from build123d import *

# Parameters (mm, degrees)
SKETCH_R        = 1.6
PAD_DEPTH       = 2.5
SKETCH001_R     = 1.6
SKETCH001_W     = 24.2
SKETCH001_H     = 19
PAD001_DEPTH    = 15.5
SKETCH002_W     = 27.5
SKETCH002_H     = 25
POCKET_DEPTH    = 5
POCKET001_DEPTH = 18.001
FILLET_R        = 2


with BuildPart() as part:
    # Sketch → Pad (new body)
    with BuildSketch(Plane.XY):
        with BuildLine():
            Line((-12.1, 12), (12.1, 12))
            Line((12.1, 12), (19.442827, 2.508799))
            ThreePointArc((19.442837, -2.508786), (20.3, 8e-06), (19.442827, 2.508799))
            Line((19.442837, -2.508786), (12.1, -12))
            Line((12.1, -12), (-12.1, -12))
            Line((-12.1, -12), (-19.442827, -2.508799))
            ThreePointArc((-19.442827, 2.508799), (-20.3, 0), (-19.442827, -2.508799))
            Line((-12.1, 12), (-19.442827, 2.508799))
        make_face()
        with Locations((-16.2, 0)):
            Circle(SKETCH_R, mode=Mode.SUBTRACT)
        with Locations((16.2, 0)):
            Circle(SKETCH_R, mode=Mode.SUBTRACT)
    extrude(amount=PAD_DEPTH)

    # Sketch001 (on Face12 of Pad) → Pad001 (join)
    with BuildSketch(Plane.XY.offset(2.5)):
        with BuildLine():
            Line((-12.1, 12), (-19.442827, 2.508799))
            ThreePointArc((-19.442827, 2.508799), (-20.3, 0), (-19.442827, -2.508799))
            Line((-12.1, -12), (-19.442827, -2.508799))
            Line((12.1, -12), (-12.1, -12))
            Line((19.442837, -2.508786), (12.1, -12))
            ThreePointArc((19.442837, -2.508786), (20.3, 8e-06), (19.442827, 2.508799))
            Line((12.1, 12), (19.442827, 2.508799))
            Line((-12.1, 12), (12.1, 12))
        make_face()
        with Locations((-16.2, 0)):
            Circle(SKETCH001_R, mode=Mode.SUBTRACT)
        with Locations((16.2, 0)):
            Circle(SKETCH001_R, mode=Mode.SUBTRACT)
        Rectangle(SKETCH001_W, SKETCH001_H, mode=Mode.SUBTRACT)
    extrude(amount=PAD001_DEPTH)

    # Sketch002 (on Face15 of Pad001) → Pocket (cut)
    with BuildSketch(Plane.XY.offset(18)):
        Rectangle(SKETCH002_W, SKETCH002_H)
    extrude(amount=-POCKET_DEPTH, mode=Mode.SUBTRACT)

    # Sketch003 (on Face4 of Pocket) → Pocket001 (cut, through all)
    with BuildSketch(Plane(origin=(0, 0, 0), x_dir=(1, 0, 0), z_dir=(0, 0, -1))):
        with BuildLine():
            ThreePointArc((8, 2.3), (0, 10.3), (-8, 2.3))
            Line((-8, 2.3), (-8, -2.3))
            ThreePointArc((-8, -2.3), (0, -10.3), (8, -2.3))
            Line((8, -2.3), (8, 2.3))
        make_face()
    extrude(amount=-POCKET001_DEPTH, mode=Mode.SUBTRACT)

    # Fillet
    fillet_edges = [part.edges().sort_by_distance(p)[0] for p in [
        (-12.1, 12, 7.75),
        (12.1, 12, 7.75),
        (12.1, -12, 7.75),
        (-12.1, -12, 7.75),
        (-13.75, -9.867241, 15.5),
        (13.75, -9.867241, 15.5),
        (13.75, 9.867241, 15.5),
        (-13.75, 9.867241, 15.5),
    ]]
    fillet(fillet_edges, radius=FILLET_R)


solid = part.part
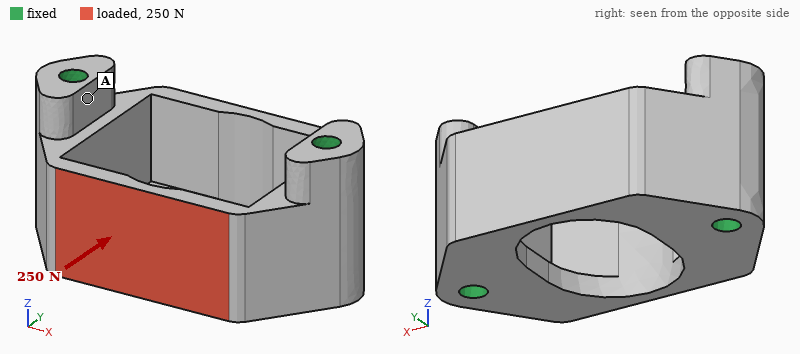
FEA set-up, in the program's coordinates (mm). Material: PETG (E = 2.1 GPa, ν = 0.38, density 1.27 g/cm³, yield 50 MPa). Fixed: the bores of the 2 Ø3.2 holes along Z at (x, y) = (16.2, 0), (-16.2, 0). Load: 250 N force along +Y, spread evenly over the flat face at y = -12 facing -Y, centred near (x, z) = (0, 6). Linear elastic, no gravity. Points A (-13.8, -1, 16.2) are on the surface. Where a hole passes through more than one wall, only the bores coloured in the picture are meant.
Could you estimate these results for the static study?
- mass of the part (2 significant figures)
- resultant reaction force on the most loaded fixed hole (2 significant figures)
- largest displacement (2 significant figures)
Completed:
6.5 g
170 N
0.58 mm
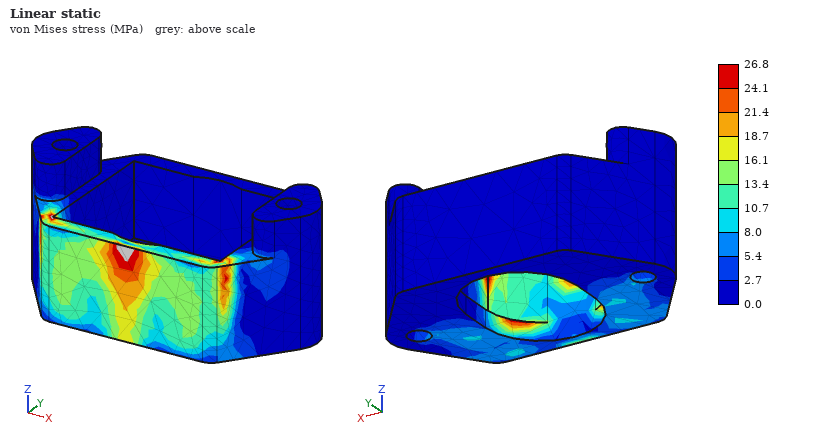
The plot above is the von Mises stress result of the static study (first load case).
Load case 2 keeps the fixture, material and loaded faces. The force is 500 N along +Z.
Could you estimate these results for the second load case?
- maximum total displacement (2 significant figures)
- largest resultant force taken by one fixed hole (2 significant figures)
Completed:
0.53 mm
250 N
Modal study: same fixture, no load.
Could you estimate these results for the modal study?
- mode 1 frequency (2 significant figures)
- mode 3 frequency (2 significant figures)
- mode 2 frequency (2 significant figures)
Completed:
5000 Hz
6100 Hz
5000 Hz
